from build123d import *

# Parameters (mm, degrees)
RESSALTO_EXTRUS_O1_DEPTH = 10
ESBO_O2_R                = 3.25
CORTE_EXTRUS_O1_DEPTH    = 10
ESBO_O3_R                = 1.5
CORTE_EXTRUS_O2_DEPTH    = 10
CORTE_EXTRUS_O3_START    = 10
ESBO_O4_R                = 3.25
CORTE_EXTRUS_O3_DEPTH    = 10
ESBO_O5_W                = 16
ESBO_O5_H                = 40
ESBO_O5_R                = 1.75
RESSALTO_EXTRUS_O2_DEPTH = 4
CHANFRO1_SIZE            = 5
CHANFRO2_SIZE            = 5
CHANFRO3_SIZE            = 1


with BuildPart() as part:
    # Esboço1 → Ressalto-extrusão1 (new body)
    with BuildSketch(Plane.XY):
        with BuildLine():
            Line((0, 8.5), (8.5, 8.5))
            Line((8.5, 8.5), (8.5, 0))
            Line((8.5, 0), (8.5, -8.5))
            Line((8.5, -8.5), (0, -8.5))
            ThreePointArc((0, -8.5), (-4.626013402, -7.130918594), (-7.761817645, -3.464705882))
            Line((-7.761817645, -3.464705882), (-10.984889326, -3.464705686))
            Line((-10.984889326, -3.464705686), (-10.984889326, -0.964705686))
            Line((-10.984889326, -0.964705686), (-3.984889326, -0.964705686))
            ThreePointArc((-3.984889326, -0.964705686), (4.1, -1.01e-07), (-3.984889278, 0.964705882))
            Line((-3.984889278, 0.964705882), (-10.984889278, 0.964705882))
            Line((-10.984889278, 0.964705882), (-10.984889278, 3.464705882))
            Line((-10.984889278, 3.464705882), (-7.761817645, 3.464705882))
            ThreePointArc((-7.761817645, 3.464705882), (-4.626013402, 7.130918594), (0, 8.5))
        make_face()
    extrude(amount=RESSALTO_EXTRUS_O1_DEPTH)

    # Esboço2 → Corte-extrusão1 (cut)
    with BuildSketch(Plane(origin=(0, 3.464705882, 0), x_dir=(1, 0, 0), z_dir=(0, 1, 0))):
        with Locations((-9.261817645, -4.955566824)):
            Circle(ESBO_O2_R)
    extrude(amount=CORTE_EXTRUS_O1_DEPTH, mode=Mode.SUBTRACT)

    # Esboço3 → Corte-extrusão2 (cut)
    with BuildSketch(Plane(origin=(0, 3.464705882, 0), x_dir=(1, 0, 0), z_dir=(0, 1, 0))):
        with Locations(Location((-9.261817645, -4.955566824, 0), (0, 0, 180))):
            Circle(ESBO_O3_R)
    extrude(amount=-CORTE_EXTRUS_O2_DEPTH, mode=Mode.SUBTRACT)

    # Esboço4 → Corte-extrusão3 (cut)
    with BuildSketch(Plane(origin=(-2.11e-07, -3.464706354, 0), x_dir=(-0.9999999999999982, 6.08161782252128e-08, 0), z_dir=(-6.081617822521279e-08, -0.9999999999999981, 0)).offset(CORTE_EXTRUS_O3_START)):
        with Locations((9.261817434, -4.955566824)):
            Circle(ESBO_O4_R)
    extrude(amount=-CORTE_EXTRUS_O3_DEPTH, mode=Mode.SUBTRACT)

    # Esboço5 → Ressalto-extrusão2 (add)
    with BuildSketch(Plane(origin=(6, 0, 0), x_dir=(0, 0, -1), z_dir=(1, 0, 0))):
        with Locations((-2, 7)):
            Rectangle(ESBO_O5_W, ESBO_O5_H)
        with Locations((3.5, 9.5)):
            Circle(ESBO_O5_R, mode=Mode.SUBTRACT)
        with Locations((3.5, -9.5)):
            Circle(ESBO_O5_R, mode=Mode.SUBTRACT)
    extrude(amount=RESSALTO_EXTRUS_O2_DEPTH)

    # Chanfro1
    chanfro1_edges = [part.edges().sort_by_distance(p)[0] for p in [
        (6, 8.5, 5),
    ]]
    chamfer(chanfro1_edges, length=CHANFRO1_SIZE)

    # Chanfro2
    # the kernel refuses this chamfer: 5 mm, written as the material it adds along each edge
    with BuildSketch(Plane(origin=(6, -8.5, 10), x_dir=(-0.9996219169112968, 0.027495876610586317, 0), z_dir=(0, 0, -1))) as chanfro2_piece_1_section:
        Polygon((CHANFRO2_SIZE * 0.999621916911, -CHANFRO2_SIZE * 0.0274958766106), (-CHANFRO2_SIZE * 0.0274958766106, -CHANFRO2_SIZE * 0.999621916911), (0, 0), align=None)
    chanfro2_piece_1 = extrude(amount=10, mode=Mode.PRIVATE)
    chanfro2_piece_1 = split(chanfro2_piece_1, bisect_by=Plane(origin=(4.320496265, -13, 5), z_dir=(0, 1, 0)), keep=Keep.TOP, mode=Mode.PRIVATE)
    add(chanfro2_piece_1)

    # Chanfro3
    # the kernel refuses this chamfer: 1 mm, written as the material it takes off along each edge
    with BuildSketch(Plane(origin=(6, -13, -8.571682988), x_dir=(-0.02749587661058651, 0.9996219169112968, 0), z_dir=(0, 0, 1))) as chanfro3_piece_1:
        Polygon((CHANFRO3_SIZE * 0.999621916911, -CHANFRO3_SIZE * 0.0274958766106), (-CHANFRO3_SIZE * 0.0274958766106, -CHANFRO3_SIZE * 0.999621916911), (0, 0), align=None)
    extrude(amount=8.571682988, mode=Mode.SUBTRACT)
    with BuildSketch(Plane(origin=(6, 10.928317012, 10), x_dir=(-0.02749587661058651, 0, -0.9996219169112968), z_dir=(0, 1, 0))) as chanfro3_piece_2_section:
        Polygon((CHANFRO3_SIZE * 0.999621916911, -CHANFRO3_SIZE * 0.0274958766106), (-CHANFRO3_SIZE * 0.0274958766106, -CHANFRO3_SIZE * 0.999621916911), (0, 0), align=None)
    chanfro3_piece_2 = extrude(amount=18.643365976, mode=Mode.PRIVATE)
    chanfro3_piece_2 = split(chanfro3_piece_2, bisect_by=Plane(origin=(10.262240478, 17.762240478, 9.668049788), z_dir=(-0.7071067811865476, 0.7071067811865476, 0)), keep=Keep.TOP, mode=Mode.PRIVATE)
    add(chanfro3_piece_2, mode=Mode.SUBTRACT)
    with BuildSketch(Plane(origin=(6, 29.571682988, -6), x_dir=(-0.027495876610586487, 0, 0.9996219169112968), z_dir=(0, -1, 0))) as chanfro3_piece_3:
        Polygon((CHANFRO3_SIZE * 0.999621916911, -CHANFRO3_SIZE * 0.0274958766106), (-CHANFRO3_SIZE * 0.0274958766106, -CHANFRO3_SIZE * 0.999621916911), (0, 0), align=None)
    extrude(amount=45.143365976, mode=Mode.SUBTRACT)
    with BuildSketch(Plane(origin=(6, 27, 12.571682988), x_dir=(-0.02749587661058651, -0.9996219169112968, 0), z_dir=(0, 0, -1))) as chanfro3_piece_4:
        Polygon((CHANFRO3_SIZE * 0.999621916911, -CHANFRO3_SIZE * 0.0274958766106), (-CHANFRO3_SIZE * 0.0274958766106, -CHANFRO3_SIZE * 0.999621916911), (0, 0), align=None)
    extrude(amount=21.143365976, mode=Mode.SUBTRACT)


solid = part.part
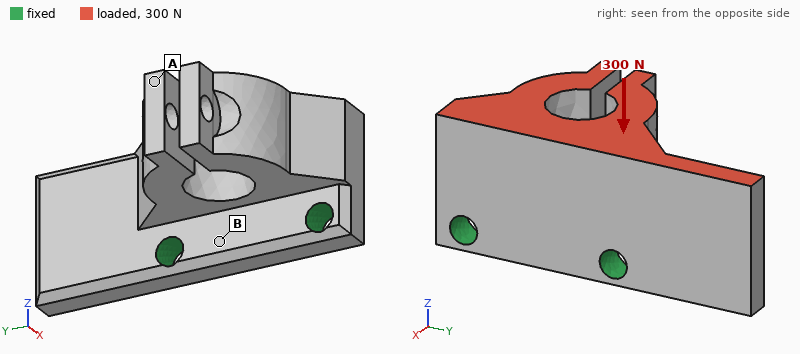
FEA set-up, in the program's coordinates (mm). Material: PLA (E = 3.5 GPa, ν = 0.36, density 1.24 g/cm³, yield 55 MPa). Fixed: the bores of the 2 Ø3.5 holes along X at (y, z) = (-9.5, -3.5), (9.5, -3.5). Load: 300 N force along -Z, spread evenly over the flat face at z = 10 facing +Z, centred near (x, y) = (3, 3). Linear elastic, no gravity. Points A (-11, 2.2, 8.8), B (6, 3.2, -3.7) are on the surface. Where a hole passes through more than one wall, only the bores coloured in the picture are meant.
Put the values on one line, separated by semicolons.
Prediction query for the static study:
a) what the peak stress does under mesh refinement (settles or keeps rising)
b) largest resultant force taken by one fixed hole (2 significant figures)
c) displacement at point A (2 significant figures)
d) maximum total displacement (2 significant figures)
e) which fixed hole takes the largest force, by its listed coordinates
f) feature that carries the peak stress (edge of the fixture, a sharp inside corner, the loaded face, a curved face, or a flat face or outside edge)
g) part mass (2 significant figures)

keeps rising; 190 N; 0.36 mm; 0.38 mm; (9.5, -3.5); edge of the fixture; 5.4 g
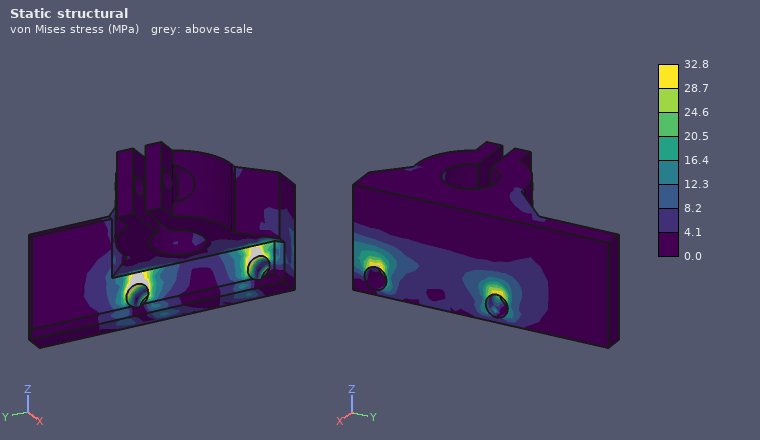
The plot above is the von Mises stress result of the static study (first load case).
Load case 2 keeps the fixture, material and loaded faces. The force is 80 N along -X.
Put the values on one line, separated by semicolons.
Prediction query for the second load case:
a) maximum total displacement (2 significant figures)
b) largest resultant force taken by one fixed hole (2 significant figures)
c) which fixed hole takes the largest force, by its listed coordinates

0.22 mm; 50 N; (9.5, -3.5)
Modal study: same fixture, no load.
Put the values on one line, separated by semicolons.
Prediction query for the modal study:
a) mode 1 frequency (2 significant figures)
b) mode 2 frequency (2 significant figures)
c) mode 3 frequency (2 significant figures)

2400 Hz; 3400 Hz; 4900 Hz
